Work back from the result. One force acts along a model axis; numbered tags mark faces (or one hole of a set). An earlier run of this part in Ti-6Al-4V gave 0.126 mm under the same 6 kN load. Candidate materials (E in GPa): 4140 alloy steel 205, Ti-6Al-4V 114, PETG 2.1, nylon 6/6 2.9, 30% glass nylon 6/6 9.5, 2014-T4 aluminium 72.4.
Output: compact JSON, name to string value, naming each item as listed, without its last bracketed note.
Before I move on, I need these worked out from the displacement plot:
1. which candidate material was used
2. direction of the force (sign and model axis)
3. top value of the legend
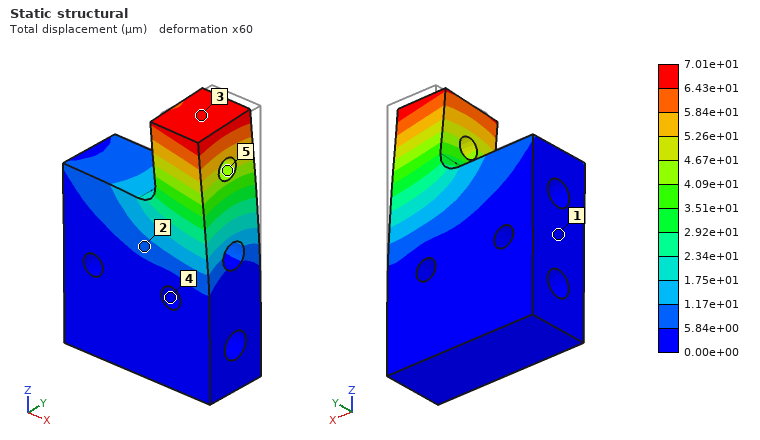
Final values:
{"which candidate material was used": "4140 alloy steel", "direction of the force": "-Y", "top value of the legend": "7.01e+01 µm"}
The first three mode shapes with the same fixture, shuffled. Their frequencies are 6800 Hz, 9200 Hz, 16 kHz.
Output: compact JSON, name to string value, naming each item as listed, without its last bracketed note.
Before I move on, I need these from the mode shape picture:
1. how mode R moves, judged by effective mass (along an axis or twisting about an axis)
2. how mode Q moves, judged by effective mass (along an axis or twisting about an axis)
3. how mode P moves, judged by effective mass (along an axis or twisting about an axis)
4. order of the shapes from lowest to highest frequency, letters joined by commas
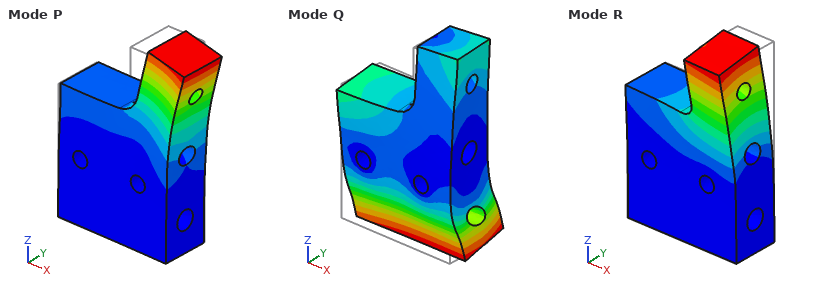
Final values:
{"how mode R moves, judged by effective mass": "along Y", "how mode Q moves, judged by effective mass": "along Y", "how mode P moves, judged by effective mass": "along X", "order of the shapes from lowest to highest frequency, letters joined by commas": "R, P, Q"}
